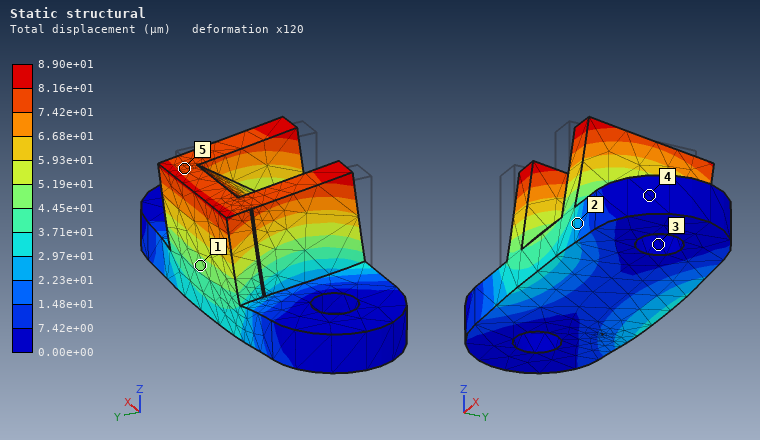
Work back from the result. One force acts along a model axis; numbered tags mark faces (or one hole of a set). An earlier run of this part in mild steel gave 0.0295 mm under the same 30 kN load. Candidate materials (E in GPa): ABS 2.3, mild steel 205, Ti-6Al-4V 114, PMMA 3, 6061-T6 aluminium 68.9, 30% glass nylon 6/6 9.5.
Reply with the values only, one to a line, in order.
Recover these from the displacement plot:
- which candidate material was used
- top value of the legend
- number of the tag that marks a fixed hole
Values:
6061-T6 aluminium
8.90e+01 µm
3
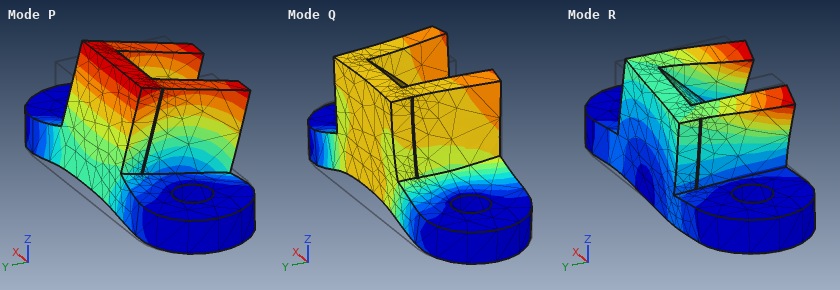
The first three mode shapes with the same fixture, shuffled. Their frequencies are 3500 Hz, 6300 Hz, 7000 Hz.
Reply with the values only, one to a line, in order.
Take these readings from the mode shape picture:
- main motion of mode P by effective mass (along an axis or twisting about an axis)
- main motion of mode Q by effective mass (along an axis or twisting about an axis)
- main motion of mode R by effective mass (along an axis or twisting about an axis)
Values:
along Y
along Z
along X
